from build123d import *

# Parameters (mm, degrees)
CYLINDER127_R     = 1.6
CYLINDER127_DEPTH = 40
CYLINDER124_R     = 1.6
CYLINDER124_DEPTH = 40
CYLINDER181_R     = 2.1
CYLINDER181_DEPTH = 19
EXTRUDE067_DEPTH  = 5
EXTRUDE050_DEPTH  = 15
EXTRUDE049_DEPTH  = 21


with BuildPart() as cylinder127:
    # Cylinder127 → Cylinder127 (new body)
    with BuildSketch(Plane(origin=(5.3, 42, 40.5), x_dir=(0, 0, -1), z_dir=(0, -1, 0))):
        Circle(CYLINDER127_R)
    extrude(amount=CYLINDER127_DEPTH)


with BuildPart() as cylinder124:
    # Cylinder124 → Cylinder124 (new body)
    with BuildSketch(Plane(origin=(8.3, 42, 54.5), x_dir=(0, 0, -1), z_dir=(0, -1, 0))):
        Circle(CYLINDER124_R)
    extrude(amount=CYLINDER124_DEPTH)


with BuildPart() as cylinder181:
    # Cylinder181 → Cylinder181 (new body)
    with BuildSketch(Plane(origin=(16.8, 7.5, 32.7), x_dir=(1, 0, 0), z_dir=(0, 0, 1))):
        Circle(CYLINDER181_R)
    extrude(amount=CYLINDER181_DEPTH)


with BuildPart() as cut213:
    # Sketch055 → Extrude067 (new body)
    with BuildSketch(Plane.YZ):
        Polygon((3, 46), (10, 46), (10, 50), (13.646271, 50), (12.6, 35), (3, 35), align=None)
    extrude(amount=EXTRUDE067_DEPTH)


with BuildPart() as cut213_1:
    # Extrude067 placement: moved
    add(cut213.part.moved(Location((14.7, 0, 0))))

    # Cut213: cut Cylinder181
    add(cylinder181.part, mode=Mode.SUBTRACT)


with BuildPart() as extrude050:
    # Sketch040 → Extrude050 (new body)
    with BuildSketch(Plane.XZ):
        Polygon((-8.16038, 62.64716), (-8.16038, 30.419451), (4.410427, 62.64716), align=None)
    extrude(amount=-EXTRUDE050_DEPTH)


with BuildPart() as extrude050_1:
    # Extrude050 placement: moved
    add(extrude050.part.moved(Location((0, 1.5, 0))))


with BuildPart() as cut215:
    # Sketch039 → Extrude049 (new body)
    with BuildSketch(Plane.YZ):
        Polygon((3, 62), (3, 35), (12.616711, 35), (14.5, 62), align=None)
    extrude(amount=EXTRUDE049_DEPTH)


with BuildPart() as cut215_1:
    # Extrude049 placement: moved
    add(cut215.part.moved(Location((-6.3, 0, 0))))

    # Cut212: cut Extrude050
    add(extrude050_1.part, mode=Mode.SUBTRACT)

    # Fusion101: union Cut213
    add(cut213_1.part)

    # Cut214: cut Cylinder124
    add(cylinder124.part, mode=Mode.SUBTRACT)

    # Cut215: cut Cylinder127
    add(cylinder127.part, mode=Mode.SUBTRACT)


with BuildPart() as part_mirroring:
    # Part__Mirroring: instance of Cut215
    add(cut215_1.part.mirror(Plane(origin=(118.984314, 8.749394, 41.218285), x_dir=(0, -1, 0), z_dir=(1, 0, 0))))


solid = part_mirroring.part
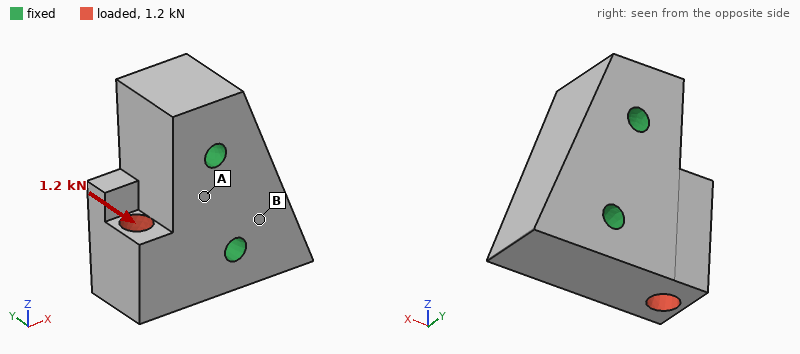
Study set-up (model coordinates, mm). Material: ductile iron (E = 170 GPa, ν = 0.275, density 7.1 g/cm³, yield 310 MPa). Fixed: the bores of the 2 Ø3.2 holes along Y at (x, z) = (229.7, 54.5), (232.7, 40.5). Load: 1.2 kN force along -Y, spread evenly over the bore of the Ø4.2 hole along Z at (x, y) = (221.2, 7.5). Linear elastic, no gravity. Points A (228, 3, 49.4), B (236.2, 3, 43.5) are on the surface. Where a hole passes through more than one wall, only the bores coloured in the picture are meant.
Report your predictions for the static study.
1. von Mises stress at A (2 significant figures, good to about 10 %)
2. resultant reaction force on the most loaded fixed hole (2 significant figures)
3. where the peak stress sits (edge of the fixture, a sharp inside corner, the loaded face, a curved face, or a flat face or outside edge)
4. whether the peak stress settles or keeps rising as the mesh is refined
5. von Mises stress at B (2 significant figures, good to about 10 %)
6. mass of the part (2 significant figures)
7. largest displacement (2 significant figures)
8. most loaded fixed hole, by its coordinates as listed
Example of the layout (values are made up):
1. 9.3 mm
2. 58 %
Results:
1. 24 MPa
2. 900 N
3. edge of the fixture
4. keeps rising
5. 8.7 MPa
6. 34 g
7. 8.1 µm
8. (232.7, 40.5)
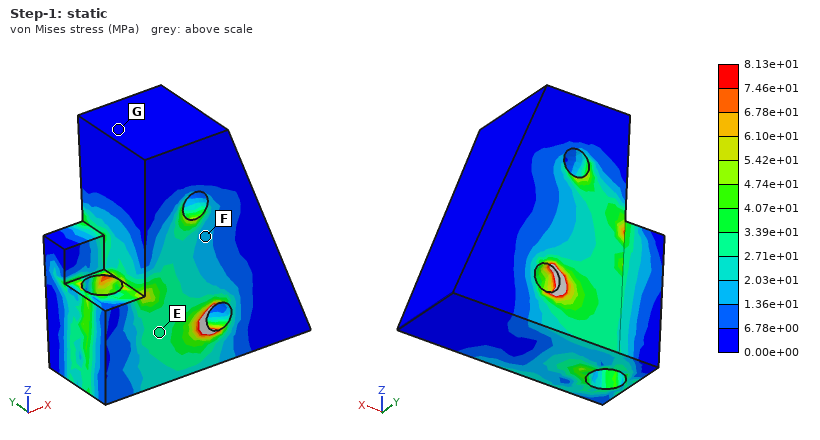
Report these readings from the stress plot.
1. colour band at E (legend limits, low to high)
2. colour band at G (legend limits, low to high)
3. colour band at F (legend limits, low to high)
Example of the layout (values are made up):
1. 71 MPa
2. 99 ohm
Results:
1. 2.71e+01 to 3.39e+01 MPa
2. 0.00e+00 to 6.78e+00 MPa
3. 1.36e+01 to 2.03e+01 MPa
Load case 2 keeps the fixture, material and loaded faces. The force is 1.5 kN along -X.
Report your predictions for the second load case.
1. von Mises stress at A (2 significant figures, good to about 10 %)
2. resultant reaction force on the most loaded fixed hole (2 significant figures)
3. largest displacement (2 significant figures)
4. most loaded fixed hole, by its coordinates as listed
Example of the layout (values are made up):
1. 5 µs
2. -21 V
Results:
1. 3.8 MPa
2. 1.4 kN
3. 2.8 µm
4. (232.7, 40.5)
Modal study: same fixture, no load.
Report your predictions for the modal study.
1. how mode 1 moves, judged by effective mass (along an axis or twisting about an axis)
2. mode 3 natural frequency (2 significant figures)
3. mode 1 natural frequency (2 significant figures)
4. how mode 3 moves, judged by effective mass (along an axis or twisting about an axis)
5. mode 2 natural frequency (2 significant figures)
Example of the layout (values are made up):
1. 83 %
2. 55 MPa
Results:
1. along Y
2. 54 kHz
3. 34 kHz
4. along Y
5. 49 kHz
